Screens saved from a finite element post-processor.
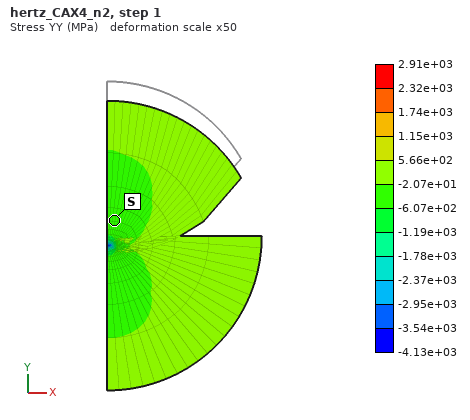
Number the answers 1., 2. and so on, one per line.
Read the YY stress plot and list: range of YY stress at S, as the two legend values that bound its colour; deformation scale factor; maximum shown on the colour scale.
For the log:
1. -6.07e+02 to -2.07e+01 MPa
2. 50
3. 2.91e+03 MPa
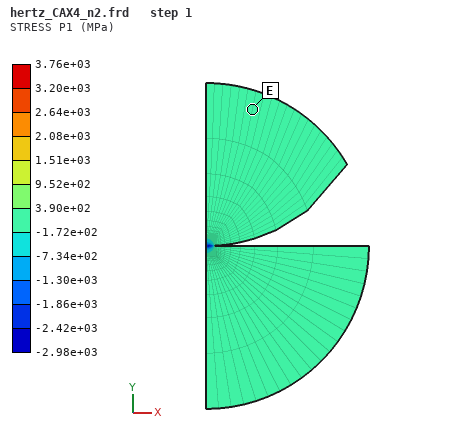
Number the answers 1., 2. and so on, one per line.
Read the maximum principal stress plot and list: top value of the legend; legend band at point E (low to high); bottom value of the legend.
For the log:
1. 3.76e+03 MPa
2. -1.72e+02 to 3.90e+02 MPa
3. -2.98e+03 MPa
